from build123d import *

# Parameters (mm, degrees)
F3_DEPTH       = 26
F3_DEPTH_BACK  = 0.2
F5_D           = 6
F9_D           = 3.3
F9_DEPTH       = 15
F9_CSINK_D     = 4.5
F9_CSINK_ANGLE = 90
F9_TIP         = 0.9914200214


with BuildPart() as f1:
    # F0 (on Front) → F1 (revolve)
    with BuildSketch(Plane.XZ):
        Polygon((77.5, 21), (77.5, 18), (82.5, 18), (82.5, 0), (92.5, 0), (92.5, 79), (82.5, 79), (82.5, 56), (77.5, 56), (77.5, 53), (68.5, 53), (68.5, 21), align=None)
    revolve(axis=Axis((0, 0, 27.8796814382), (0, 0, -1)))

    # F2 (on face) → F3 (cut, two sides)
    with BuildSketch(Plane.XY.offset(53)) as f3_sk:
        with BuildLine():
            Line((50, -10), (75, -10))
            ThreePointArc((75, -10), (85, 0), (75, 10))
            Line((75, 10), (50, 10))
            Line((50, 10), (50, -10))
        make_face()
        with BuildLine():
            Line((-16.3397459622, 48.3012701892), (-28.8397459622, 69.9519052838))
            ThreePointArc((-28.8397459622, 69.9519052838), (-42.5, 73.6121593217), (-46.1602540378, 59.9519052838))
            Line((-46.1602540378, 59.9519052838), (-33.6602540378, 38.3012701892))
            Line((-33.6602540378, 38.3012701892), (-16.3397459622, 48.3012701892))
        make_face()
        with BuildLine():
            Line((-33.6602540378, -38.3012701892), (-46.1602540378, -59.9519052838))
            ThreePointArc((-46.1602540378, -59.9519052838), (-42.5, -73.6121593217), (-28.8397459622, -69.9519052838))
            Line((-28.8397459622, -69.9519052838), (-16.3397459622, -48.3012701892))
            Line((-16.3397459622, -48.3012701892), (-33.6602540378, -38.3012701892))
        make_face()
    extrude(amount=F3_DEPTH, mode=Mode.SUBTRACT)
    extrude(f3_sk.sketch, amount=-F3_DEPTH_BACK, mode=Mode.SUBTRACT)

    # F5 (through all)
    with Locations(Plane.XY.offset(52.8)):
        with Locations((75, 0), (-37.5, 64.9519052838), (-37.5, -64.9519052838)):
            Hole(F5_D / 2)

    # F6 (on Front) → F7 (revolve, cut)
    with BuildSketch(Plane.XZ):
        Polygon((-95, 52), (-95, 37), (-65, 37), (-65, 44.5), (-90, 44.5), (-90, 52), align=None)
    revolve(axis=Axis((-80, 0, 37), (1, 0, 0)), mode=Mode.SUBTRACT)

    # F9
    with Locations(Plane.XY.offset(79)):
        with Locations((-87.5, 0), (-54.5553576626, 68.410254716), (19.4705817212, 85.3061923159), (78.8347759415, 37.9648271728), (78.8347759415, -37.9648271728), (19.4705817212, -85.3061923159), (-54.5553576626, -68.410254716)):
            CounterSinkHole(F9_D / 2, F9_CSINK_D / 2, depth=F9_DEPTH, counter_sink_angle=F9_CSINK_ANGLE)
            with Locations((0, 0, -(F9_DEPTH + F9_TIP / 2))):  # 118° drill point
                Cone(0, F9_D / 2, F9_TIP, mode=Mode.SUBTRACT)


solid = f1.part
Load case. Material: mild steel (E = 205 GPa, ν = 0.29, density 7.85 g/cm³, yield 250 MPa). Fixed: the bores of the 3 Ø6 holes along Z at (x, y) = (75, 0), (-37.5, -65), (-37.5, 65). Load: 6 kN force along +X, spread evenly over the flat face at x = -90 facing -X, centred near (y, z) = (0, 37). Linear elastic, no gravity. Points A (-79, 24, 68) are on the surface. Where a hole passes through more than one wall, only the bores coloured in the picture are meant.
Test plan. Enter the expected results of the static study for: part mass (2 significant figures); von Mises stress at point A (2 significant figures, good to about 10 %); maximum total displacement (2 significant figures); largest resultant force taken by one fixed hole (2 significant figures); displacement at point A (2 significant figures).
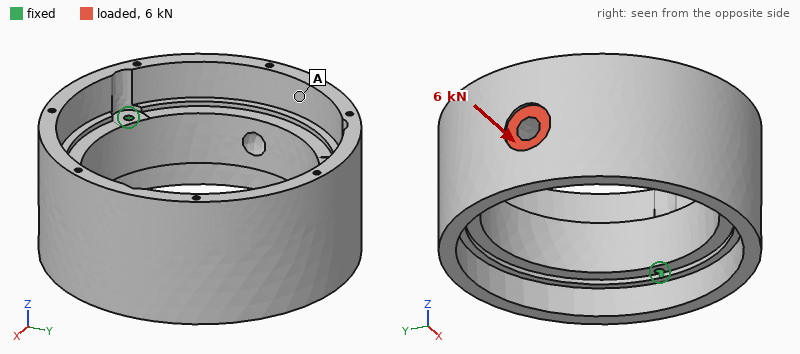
5.1 kg
2.4 MPa
6.1 µm
4.5 kN
2.8 µm
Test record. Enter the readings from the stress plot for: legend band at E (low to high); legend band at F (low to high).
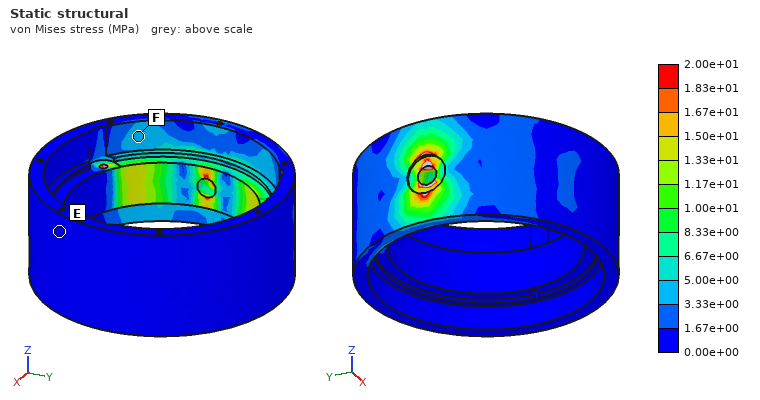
0.00e+00 to 1.67e+00 MPa
3.33e+00 to 5.00e+00 MPa
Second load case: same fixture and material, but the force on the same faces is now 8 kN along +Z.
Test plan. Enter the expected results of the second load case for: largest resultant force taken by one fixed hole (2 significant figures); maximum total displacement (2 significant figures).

4.6 kN
28 µm
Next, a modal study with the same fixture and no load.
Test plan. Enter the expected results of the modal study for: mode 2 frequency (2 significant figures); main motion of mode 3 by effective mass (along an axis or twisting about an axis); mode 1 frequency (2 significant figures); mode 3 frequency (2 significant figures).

3400 Hz
twisting about Z
3400 Hz
4700 Hz
